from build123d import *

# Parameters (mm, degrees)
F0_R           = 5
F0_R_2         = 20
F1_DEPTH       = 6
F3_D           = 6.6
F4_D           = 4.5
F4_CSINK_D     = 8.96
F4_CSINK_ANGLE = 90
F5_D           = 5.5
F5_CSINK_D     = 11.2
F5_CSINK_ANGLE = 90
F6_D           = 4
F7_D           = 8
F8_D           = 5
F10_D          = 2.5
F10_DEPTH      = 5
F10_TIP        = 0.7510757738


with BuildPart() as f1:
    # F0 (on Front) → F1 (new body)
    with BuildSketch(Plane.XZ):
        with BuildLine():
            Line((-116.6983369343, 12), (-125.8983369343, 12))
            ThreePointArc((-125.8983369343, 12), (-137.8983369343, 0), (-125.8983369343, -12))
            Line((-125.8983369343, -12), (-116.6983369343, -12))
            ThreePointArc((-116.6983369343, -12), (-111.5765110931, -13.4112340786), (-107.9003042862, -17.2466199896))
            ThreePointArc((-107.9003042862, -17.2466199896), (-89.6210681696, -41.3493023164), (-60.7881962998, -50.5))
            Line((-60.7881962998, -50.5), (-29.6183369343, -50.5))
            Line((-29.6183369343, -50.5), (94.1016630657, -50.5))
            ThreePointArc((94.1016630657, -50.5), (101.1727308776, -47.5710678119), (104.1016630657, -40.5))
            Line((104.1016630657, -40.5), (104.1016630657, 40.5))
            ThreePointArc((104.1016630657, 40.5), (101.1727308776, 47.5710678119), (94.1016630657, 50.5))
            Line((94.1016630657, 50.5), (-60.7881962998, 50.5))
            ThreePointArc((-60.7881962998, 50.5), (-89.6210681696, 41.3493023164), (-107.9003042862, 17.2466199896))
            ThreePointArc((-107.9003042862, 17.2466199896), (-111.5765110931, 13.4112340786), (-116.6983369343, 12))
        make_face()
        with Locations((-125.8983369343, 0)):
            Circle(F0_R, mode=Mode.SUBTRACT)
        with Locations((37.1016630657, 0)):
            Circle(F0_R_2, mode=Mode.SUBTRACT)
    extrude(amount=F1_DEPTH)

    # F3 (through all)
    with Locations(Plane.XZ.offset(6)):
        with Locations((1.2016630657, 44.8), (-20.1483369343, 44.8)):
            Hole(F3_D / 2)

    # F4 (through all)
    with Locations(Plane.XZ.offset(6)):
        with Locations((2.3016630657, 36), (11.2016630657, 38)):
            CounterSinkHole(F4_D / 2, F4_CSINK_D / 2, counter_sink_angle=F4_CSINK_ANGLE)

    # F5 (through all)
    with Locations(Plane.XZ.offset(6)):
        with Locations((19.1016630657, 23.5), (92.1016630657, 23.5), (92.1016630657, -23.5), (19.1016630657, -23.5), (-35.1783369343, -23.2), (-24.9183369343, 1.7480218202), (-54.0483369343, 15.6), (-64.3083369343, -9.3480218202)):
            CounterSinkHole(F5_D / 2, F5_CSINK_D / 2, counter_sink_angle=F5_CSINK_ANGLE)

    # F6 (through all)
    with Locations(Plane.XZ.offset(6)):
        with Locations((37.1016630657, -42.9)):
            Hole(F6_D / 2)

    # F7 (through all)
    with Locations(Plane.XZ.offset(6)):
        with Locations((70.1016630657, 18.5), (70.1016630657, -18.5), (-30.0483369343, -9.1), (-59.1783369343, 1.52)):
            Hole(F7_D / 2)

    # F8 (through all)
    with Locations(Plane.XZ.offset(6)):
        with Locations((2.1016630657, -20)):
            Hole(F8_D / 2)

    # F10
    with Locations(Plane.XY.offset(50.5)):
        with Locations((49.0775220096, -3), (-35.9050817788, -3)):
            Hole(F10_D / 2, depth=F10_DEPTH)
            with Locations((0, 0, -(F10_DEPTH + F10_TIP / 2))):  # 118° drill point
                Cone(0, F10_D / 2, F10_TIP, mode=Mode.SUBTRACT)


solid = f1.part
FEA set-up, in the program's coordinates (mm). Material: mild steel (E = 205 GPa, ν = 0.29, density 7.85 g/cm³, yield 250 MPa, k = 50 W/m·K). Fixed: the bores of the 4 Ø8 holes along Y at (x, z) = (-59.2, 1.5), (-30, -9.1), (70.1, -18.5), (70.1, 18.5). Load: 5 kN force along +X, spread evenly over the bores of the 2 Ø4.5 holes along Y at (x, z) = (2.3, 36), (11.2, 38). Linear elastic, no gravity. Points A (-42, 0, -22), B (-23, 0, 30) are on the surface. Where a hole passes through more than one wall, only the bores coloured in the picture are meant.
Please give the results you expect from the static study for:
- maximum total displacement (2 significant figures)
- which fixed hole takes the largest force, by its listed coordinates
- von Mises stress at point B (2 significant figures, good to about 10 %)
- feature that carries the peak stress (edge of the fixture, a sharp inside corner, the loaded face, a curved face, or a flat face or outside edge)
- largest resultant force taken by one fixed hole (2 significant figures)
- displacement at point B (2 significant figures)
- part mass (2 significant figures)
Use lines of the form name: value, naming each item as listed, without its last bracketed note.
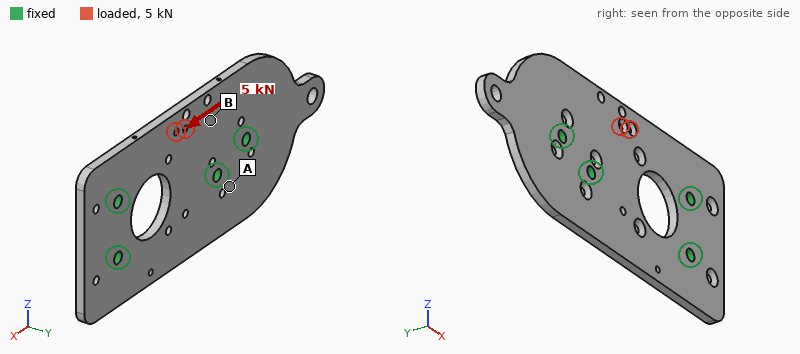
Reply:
maximum total displacement: 9.0 µm
which fixed hole takes the largest force, by its listed coordinates: (70.1, 18.5)
von Mises stress at point B: 13 MPa
feature that carries the peak stress: the loaded face
largest resultant force taken by one fixed hole: 2.4 kN
displacement at point B: 5.4 µm
part mass: 900 g
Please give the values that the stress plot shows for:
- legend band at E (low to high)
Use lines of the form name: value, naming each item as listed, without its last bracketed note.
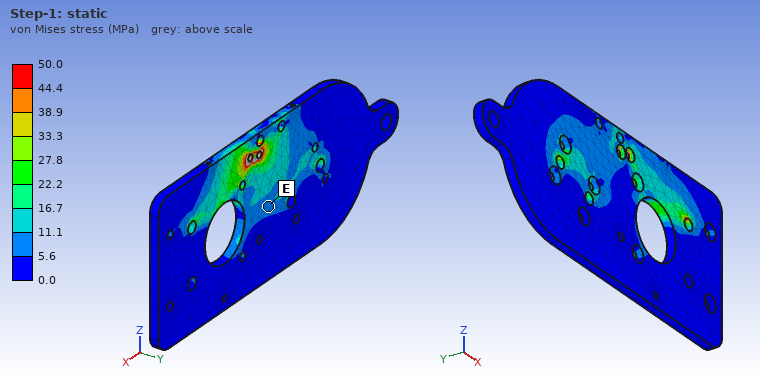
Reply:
legend band at E: 5.6 to 11.1 MPa
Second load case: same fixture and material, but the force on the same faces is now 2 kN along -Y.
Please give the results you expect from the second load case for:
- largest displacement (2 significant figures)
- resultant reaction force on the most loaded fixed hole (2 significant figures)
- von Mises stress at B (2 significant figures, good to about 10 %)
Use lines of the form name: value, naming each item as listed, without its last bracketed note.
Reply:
largest displacement: 0.24 mm
resultant reaction force on the most loaded fixed hole: 1000 N
von Mises stress at B: 36 MPa
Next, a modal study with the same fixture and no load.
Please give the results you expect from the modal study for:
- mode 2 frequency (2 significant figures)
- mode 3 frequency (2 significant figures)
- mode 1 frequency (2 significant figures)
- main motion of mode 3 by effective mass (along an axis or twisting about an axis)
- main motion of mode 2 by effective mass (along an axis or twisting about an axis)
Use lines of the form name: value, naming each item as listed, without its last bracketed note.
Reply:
mode 2 frequency: 1700 Hz
mode 3 frequency: 2100 Hz
mode 1 frequency: 1300 Hz
main motion of mode 3 by effective mass: along Y
main motion of mode 2 by effective mass: along Y
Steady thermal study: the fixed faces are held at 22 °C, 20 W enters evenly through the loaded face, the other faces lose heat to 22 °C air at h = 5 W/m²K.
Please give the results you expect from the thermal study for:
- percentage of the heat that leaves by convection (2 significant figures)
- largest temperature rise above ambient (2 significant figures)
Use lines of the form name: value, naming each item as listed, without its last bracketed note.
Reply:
percentage of the heat that leaves by convection: 9.3 %
largest temperature rise above ambient: 57 K
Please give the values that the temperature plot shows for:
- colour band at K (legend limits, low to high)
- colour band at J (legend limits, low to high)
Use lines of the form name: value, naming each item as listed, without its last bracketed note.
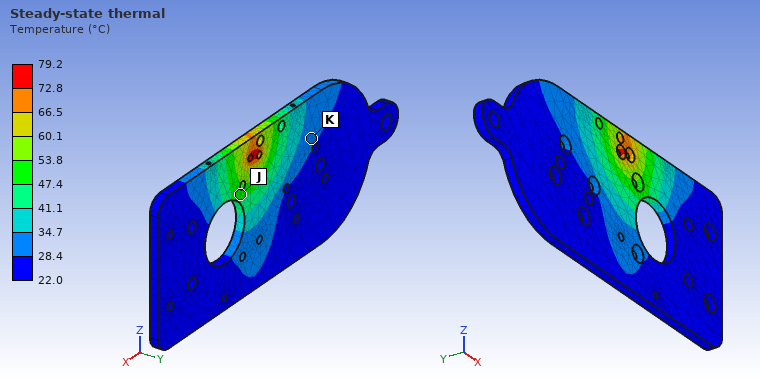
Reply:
colour band at K: 28.4 to 34.7 °C
colour band at J: 47.4 to 53.8 °C
